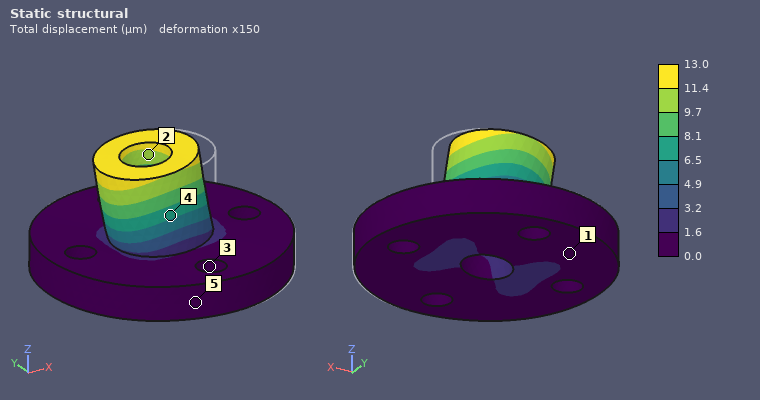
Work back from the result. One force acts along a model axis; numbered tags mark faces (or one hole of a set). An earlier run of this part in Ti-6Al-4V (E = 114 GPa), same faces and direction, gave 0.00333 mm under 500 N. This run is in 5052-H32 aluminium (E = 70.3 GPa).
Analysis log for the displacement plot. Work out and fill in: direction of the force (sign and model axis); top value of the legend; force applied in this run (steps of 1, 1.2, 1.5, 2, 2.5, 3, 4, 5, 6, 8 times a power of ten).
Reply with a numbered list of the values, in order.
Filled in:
1. -X
2. 13.0 µm
3. 1.2 kN
